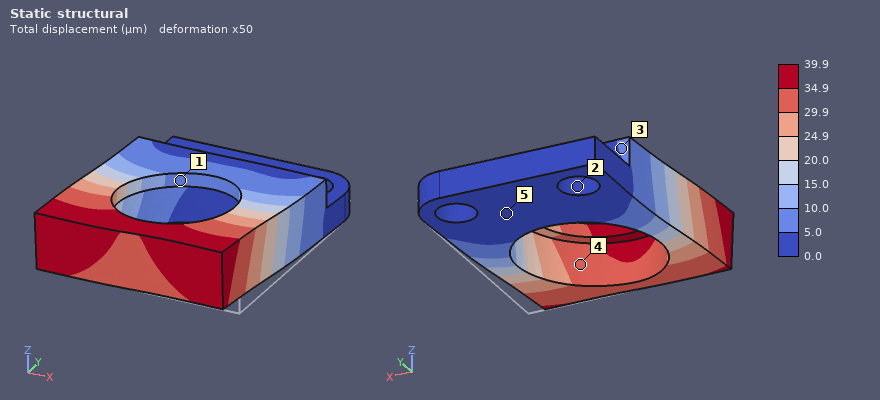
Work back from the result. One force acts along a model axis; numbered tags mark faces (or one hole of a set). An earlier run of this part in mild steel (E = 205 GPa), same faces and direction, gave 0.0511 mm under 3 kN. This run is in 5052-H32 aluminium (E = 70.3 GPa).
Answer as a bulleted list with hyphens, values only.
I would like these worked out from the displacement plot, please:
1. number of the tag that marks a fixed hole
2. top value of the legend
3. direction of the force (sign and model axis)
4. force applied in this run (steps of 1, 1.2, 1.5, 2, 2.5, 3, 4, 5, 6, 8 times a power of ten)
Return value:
- 2
- 39.9 µm
- -X
- 800 N
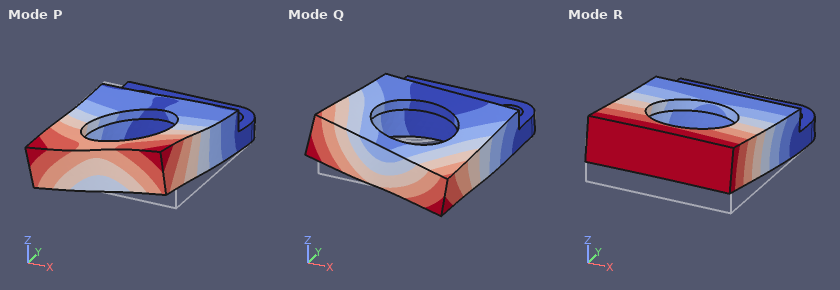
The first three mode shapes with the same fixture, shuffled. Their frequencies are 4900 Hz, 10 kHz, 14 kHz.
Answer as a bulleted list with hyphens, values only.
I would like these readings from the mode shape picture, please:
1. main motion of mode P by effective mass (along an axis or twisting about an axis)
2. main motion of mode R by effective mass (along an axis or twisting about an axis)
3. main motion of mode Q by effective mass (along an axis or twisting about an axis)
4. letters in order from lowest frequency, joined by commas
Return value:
- along X
- along Z
- along X
- R, Q, P
